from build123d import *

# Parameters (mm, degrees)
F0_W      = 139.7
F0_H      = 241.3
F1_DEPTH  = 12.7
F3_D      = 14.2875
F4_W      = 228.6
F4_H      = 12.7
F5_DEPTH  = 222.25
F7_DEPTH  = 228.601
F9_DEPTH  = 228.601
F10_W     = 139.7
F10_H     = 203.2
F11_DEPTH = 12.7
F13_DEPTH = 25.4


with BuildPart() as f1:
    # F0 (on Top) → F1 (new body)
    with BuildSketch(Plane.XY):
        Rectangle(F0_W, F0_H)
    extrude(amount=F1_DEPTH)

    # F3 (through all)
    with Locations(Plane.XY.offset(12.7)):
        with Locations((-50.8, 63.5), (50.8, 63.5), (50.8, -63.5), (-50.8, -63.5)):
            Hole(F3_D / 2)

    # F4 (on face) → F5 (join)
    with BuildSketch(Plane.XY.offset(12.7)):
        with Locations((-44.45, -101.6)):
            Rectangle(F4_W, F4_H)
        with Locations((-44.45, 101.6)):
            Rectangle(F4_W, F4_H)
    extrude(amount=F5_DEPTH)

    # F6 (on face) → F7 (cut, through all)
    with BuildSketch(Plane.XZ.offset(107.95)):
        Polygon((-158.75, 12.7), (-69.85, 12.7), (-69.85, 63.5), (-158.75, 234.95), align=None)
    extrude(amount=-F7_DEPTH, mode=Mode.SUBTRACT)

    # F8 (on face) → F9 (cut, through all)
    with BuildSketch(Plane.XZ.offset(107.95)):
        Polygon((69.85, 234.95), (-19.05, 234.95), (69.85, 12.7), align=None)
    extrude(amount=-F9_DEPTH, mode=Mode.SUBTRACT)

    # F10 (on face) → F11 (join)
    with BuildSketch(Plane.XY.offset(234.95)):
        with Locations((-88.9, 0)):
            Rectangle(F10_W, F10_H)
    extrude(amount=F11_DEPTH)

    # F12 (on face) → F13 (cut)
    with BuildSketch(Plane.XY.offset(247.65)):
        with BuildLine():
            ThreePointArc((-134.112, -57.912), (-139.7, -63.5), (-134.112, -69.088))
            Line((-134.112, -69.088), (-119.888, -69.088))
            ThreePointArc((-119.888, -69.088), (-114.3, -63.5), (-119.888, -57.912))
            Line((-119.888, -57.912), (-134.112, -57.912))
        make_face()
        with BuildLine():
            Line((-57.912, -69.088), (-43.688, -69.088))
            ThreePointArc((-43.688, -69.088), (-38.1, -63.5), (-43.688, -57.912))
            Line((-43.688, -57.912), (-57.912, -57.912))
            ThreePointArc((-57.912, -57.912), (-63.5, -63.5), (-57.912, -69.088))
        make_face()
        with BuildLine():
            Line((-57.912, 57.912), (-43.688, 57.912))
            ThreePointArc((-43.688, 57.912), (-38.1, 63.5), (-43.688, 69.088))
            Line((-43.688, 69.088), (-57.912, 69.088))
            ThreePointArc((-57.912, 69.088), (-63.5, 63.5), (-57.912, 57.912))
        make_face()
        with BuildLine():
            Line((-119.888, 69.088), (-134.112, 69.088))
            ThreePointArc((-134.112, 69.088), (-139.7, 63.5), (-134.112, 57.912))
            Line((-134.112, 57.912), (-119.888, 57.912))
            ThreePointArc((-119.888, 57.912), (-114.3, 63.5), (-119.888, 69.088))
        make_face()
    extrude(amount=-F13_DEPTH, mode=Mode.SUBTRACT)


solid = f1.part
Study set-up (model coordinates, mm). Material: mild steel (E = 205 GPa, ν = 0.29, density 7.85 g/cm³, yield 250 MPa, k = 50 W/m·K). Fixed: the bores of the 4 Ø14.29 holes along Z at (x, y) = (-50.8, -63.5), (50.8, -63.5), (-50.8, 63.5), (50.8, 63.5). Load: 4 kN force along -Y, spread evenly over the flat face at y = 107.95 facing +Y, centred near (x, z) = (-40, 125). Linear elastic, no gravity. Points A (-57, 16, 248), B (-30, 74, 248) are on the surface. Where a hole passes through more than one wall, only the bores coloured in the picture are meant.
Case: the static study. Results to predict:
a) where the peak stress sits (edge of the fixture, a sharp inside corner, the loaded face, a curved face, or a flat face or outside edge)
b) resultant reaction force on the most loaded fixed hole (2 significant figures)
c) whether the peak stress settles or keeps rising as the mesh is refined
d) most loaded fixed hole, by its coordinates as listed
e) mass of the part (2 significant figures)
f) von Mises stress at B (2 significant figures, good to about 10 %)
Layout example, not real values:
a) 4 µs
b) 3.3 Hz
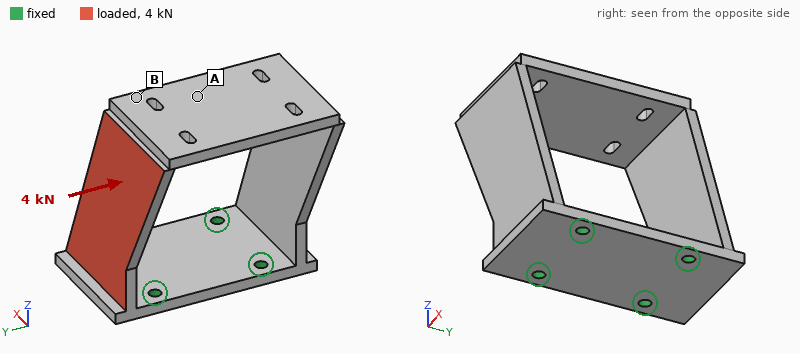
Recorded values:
a) edge of the fixture
b) 2.2 kN
c) keeps rising
d) (-50.8, 63.5)
e) 12 kg
f) 17 MPa
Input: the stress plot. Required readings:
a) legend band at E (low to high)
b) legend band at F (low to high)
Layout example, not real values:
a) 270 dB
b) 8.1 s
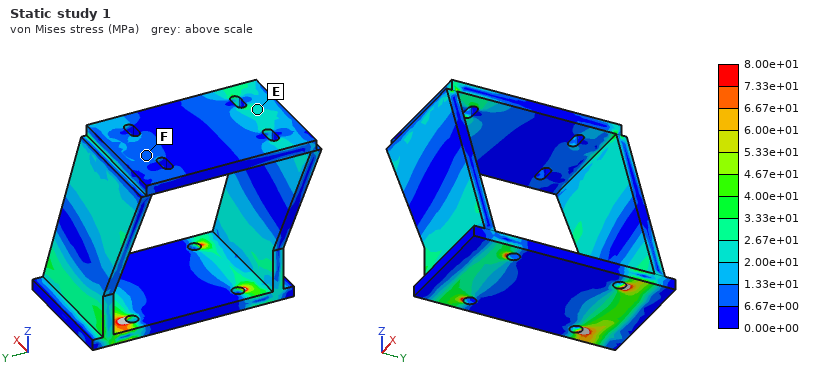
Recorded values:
a) 2.00e+01 to 2.67e+01 MPa
b) 6.67e+00 to 1.33e+01 MPa
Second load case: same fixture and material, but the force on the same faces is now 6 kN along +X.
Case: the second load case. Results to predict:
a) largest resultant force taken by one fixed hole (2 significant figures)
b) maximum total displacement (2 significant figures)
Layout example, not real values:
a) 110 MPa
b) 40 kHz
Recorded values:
a) 7.3 kN
b) 0.19 mm
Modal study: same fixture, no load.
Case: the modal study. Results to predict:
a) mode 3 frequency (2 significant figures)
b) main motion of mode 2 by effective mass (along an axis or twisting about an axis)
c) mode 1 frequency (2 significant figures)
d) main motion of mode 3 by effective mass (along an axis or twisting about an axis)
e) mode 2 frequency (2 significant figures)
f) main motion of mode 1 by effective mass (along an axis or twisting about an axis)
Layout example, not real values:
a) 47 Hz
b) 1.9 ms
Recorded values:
a) 540 Hz
b) along X
c) 140 Hz
d) twisting about Z
e) 390 Hz
f) along Y
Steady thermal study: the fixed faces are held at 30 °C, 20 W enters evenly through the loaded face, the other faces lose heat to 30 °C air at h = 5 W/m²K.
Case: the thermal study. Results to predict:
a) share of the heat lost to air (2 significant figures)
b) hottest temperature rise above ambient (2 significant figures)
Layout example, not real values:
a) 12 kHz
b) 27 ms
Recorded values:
a) 37 %
b) 18 K
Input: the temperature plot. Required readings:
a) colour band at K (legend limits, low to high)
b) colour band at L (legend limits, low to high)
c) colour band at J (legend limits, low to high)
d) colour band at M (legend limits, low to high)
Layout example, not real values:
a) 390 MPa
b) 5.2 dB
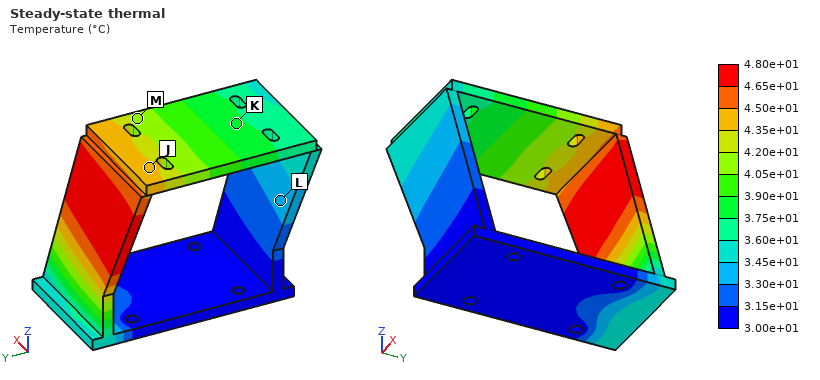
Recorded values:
a) 3.75e+01 to 3.90e+01 °C
b) 3.30e+01 to 3.45e+01 °C
c) 4.35e+01 to 4.50e+01 °C
d) 4.05e+01 to 4.20e+01 °C
